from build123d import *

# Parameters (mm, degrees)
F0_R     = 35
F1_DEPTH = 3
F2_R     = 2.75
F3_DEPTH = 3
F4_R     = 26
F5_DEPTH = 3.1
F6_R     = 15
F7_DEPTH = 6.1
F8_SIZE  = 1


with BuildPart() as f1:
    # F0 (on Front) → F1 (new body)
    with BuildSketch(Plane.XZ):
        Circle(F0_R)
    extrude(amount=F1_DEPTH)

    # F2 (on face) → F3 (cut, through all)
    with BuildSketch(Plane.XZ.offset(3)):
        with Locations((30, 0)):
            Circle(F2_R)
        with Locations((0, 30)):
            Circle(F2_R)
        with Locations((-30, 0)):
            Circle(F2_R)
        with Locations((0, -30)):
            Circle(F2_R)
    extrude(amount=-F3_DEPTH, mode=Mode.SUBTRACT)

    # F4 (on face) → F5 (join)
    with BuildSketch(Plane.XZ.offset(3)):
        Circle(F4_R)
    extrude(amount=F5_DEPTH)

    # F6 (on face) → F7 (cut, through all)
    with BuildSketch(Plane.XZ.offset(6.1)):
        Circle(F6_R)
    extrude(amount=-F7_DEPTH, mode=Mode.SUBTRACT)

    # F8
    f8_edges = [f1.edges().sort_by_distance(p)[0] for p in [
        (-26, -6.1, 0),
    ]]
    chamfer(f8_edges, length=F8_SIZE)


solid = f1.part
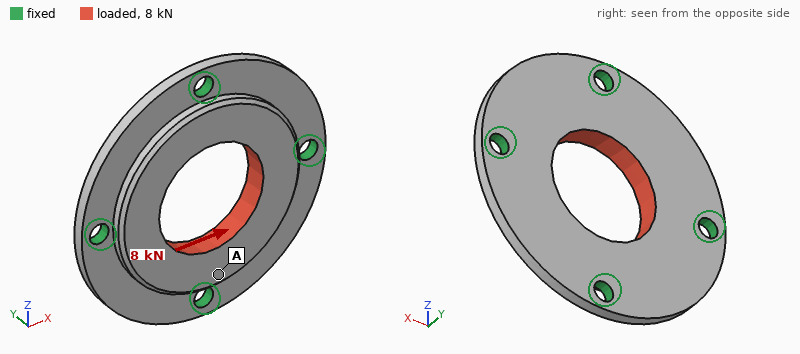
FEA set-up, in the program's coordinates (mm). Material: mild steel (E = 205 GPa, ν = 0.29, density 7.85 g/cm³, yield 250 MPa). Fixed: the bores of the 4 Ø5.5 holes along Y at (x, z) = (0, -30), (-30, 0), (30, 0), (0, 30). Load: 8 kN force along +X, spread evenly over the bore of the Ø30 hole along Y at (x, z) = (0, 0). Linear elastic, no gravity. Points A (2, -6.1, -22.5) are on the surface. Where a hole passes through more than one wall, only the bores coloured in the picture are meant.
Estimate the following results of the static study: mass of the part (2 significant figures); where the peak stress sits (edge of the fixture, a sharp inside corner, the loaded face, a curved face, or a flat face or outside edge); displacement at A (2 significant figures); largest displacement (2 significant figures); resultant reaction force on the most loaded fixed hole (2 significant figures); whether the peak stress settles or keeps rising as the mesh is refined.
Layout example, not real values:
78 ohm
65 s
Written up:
110 g
edge of the fixture
2.2 µm
4.3 µm
2.2 kN
keeps rising
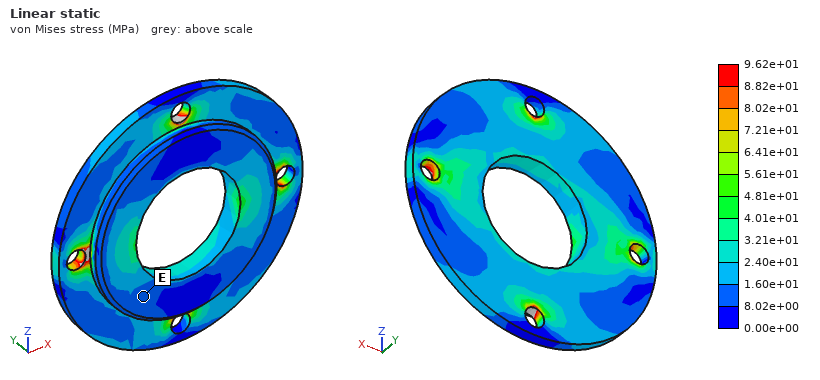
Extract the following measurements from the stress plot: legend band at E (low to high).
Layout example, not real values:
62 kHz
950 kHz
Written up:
8.02e+00 to 1.60e+01 MPa
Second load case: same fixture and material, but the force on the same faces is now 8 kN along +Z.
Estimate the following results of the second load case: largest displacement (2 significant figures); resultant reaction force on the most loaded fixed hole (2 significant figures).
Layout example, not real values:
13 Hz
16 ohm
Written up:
4.3 µm
2.2 kN
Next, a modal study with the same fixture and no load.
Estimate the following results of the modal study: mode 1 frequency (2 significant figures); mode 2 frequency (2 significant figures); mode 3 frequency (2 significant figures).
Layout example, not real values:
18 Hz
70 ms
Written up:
9800 Hz
11 kHz
11 kHz
